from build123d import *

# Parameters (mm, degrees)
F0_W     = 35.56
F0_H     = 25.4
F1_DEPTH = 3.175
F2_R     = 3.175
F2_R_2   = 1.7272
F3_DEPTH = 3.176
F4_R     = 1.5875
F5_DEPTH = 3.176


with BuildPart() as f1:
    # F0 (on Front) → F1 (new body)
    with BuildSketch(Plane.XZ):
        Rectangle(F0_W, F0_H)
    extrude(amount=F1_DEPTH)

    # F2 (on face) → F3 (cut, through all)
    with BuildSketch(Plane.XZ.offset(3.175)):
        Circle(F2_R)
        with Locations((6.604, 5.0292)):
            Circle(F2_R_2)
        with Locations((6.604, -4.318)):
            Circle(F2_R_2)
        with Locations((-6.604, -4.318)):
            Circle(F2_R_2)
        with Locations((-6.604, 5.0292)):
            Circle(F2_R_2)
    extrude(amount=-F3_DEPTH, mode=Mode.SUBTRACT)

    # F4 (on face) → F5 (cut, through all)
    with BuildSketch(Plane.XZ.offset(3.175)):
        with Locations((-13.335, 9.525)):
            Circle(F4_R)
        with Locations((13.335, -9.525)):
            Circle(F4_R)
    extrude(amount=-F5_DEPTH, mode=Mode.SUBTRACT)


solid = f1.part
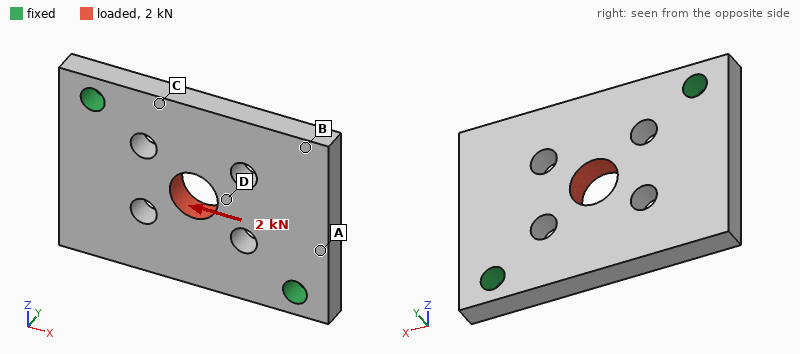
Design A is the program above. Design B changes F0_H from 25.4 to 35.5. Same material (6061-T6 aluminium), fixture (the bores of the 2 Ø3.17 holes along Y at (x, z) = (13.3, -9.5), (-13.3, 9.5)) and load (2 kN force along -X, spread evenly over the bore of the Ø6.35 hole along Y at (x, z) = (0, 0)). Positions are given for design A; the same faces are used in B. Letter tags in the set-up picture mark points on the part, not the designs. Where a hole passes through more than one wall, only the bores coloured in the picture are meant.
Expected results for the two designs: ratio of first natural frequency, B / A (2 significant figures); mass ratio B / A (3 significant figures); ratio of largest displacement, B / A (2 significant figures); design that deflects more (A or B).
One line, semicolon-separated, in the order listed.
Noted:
0.78; 1.44; 0.84; A
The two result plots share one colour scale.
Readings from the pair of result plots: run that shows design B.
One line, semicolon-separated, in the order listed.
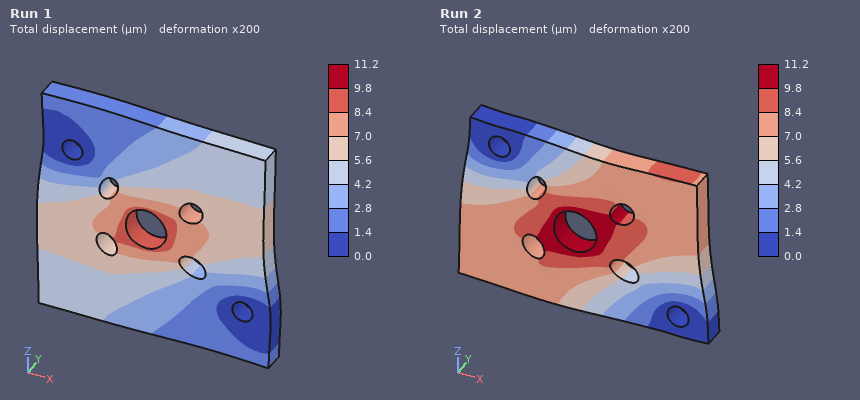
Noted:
Run 1
